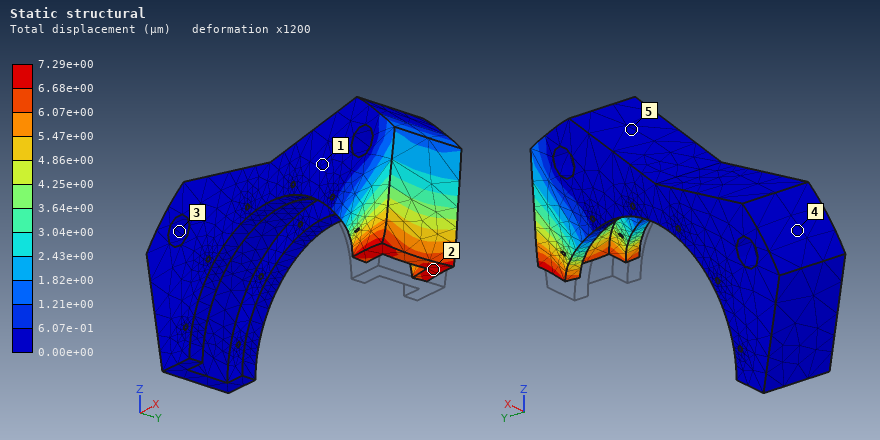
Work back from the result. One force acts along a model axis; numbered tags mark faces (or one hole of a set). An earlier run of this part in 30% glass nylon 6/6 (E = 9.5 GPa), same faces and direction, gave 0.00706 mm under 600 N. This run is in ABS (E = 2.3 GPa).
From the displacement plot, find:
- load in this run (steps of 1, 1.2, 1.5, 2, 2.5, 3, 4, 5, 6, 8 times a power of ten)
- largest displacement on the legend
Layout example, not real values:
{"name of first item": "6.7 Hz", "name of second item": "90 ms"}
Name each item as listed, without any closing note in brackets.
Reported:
{"load in this run": "150 N", "largest displacement on the legend": "7.29e+00 µm"}
